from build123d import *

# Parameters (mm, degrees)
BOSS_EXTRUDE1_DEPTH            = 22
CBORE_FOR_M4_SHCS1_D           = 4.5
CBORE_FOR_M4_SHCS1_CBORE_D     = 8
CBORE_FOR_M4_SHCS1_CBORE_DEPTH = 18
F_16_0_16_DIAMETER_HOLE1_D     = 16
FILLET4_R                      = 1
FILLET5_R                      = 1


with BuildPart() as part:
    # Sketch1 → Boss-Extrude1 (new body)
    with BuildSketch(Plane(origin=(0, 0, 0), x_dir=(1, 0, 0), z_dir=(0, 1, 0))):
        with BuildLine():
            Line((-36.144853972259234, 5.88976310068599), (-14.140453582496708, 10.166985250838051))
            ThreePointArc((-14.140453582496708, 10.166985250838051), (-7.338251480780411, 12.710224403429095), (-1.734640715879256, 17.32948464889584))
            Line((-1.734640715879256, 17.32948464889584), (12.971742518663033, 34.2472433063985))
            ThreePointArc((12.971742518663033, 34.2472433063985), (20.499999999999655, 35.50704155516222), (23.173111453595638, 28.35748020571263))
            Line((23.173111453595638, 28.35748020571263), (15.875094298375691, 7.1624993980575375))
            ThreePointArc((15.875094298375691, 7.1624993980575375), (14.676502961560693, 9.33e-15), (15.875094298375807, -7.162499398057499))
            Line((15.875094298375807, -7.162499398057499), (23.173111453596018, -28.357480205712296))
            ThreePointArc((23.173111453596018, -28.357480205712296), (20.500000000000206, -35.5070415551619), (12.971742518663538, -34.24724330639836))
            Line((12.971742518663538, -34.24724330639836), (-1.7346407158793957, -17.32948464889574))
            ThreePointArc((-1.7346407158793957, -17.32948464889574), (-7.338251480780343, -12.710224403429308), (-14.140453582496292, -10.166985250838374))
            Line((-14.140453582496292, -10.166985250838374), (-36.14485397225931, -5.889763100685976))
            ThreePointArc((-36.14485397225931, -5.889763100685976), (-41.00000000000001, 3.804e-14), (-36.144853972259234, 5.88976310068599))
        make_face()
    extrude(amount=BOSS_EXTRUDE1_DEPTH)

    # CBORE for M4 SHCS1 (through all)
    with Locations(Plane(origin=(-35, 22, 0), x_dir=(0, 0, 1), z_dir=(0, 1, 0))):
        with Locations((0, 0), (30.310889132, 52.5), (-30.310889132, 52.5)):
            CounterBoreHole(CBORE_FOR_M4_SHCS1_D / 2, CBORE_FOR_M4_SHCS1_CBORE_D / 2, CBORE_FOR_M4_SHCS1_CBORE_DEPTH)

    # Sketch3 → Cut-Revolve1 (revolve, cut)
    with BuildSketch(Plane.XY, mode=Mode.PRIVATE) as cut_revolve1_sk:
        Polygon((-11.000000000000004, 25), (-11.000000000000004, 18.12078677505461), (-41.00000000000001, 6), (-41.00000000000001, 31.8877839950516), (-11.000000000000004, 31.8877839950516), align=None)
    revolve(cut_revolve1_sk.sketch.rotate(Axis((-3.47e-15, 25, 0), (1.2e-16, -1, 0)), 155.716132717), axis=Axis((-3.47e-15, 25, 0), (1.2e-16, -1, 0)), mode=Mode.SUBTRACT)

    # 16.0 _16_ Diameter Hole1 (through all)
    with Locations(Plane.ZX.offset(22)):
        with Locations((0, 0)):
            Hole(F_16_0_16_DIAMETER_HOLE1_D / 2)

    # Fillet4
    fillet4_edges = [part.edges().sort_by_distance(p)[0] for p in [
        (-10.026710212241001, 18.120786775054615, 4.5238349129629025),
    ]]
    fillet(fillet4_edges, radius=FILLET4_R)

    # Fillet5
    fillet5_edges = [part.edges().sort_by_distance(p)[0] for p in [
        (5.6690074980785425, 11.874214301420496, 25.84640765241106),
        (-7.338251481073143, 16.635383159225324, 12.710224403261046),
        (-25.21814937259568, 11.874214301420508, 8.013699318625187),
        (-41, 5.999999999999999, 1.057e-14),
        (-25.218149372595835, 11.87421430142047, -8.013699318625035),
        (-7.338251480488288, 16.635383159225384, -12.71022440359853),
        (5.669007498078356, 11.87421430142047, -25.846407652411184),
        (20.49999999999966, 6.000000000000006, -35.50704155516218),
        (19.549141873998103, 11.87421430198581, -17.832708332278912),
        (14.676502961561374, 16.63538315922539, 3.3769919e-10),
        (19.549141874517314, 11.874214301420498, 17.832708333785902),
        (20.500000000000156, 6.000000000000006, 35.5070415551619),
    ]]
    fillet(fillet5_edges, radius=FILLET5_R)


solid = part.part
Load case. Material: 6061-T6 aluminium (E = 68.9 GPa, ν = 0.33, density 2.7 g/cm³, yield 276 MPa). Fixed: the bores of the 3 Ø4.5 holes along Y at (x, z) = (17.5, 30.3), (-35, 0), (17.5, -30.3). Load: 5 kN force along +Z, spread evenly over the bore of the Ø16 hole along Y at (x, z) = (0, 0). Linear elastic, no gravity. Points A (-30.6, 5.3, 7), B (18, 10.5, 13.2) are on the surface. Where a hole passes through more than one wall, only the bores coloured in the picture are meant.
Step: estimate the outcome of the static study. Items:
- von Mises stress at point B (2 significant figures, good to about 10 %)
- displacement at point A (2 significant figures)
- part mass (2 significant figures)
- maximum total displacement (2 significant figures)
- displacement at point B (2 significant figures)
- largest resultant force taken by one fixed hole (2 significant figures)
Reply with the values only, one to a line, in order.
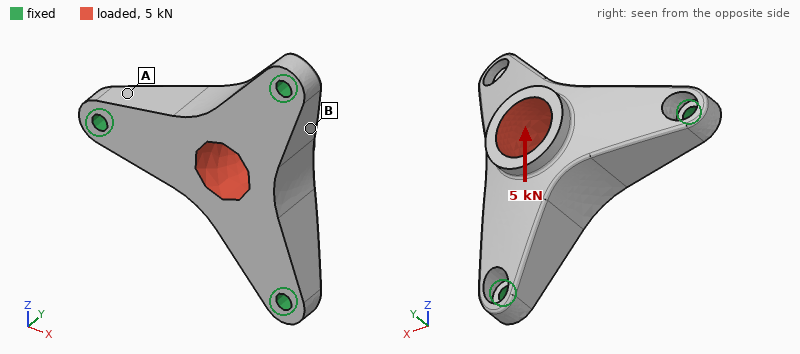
15 MPa
5.1 µm
63 g
20 µm
7.2 µm
2.6 kN
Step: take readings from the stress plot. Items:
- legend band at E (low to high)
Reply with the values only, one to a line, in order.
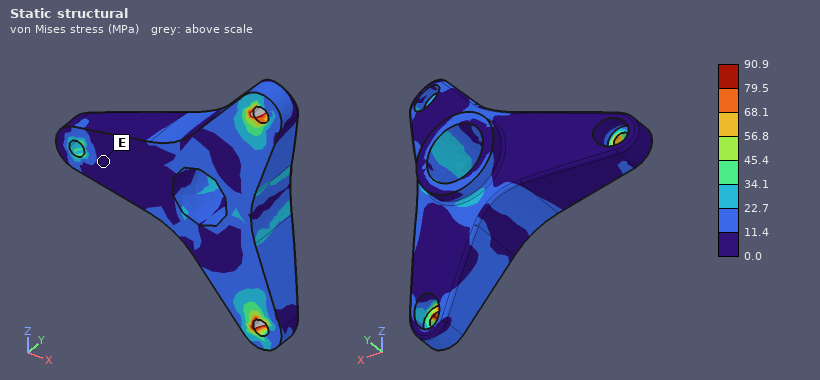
0.0 to 11.4 MPa
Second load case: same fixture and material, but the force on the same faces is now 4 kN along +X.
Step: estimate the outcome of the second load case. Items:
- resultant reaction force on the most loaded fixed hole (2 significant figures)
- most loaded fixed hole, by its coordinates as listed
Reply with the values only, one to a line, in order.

2.4 kN
(-35, 0)
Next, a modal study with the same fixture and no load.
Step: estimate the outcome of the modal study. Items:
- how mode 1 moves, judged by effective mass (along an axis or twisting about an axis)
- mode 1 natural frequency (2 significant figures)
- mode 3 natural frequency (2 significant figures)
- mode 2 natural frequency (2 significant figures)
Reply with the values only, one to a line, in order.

along Y
10 kHz
15 kHz
15 kHz
